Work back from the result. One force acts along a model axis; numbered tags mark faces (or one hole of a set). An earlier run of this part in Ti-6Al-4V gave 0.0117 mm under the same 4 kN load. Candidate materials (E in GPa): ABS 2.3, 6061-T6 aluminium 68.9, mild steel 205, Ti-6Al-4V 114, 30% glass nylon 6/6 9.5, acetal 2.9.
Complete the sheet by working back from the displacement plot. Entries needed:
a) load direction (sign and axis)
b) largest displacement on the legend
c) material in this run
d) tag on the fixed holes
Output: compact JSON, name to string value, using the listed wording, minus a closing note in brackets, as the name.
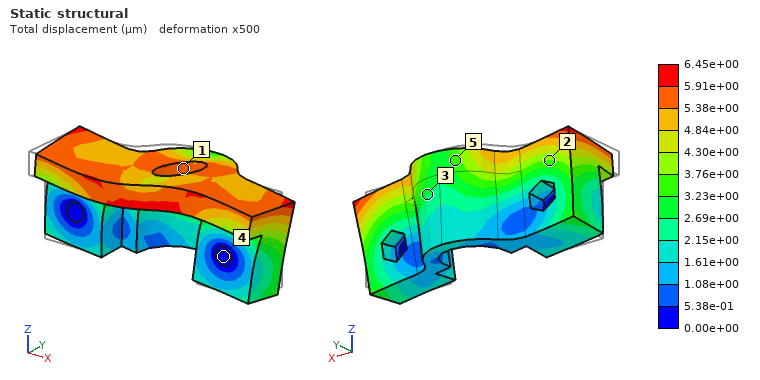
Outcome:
{"load direction": "+X", "largest displacement on the legend": "6.45e+00 µm", "material in this run": "mild steel", "tag on the fixed holes": "4"}
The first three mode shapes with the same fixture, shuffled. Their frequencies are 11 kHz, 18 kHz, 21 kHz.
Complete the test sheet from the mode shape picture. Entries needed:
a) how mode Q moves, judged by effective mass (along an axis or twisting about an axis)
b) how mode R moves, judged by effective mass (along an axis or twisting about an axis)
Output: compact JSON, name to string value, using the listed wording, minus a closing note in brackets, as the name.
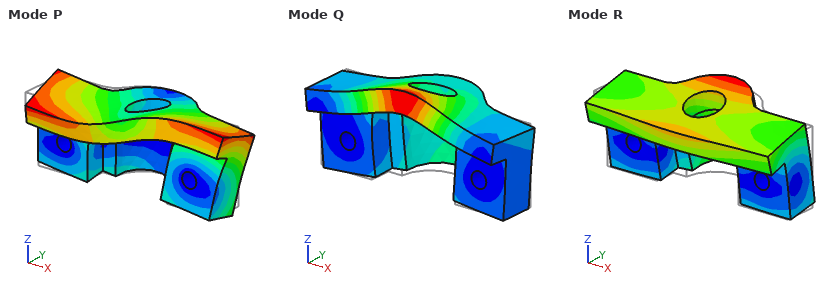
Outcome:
{"how mode Q moves, judged by effective mass": "along Z", "how mode R moves, judged by effective mass": "along Y"}
